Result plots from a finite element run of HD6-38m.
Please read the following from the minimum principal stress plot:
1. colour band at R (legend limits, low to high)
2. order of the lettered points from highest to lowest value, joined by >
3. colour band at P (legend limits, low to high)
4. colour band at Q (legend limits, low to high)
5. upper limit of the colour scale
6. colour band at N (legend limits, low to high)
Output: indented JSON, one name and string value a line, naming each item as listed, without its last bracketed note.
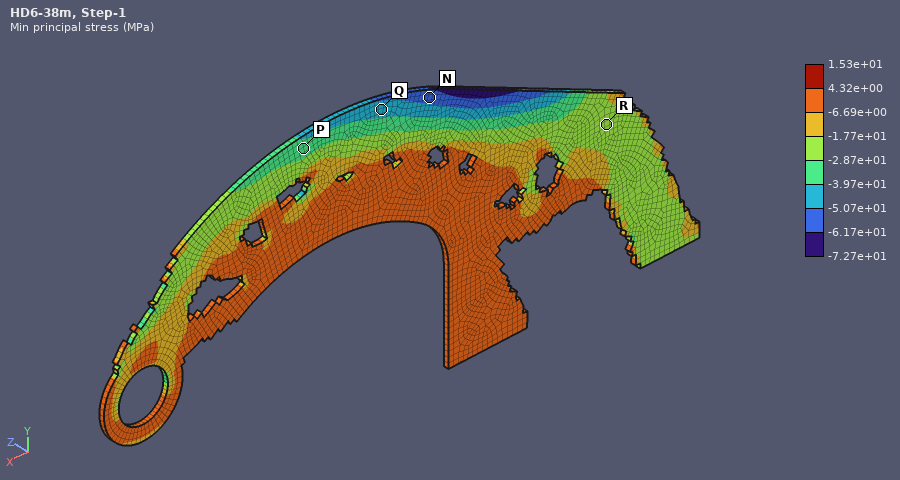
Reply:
{
  "colour band at R": "-2.87e+01 to -1.77e+01 MPa",
  "order of the lettered points from highest to lowest value, joined by >": "R > P > Q > N",
  "colour band at P": "-3.97e+01 to -2.87e+01 MPa",
  "colour band at Q": "-5.07e+01 to -3.97e+01 MPa",
  "upper limit of the colour scale": "1.53e+01 MPa",
  "colour band at N": "-6.17e+01 to -5.07e+01 MPa"
}
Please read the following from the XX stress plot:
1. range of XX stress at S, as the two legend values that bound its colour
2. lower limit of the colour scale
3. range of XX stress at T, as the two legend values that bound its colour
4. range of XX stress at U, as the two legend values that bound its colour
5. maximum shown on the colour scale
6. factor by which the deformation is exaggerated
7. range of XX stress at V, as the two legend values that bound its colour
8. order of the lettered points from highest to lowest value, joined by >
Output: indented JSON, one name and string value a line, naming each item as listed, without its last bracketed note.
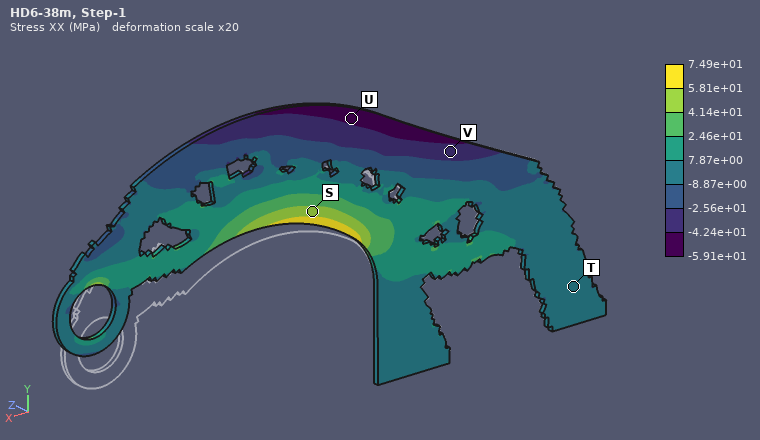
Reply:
{
  "range of XX stress at S, as the two legend values that bound its colour": "4.14e+01 to 5.81e+01 MPa",
  "lower limit of the colour scale": "-5.91e+01 MPa",
  "range of XX stress at T, as the two legend values that bound its colour": "-8.87e+00 to 7.87e+00 MPa",
  "range of XX stress at U, as the two legend values that bound its colour": "-5.91e+01 to -4.24e+01 MPa",
  "maximum shown on the colour scale": "7.49e+01 MPa",
  "factor by which the deformation is exaggerated": "20",
  "range of XX stress at V, as the two legend values that bound its colour": "-4.24e+01 to -2.56e+01 MPa",
  "order of the lettered points from highest to lowest value, joined by >": "S > T > V > U"
}
